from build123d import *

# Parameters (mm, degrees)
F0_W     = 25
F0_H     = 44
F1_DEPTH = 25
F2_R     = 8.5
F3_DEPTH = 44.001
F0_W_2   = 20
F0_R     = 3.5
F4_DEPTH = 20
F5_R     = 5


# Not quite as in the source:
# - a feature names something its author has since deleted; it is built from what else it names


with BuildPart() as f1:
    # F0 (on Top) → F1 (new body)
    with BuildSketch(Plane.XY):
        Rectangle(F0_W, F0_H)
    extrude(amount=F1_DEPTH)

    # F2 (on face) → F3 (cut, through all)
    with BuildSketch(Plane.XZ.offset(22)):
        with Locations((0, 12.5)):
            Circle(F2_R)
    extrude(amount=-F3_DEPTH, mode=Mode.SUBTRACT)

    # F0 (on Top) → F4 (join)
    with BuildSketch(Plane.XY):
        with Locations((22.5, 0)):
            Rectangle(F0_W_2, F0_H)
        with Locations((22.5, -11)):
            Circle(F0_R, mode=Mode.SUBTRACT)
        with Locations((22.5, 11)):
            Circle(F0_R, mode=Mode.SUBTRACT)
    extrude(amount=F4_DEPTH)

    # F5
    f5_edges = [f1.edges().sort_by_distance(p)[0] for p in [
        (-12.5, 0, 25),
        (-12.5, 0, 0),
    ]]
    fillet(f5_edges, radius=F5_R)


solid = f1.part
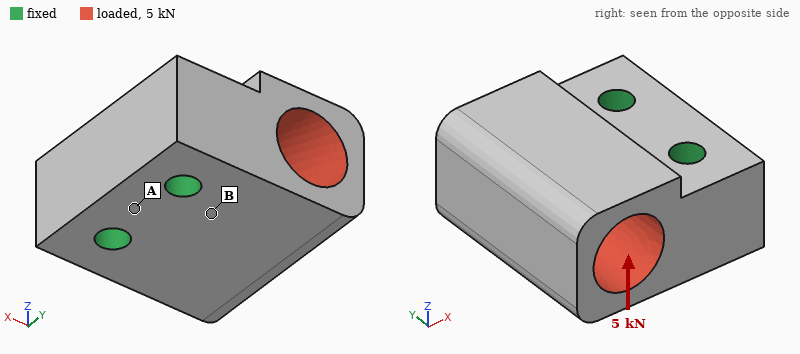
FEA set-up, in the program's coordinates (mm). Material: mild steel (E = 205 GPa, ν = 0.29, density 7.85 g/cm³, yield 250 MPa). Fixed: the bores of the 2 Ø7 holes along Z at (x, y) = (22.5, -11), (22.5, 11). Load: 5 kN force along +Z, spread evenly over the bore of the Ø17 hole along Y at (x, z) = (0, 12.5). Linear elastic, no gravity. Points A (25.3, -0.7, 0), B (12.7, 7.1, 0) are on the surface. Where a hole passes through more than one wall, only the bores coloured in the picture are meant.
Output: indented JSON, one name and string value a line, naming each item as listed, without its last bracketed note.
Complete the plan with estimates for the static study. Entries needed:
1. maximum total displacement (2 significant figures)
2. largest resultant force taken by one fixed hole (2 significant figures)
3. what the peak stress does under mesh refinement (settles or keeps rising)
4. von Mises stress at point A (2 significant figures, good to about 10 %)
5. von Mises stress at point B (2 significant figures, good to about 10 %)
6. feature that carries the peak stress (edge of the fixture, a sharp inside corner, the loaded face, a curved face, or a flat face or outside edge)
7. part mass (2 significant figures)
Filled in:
{
  "maximum total displacement": "17 µm",
  "largest resultant force taken by one fixed hole": "2.5 kN",
  "what the peak stress does under mesh refinement": "keeps rising",
  "von Mises stress at point A": "9.9 MPa",
  "von Mises stress at point B": "30 MPa",
  "feature that carries the peak stress": "edge of the fixture",
  "part mass": "260 g"
}
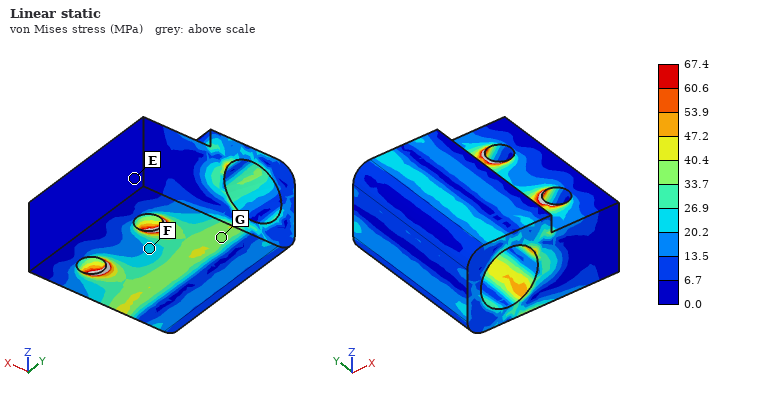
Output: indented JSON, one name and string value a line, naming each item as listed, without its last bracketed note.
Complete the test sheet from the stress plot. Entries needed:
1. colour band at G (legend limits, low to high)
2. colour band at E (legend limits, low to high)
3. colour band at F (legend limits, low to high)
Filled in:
{
  "colour band at G": "33.7 to 40.4 MPa",
  "colour band at E": "0.0 to 6.7 MPa",
  "colour band at F": "20.2 to 26.9 MPa"
}
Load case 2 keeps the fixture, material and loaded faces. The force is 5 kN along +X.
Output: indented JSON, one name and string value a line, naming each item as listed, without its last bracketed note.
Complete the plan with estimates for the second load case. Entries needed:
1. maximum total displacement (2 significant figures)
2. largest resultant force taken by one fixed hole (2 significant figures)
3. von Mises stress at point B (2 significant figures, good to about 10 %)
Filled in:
{
  "maximum total displacement": "3.8 µm",
  "largest resultant force taken by one fixed hole": "2.5 kN",
  "von Mises stress at point B": "7.6 MPa"
}
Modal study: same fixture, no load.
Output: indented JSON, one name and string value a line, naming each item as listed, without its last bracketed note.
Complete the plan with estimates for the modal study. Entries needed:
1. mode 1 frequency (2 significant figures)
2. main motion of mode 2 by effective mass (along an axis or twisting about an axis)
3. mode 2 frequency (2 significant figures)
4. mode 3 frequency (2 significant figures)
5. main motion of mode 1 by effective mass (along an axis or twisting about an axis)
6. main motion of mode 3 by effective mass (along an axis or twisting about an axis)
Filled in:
{
  "mode 1 frequency": "8400 Hz",
  "main motion of mode 2 by effective mass": "along Y",
  "mode 2 frequency": "14 kHz",
  "mode 3 frequency": "17 kHz",
  "main motion of mode 1 by effective mass": "along Z",
  "main motion of mode 3 by effective mass": "twisting about X"
}
